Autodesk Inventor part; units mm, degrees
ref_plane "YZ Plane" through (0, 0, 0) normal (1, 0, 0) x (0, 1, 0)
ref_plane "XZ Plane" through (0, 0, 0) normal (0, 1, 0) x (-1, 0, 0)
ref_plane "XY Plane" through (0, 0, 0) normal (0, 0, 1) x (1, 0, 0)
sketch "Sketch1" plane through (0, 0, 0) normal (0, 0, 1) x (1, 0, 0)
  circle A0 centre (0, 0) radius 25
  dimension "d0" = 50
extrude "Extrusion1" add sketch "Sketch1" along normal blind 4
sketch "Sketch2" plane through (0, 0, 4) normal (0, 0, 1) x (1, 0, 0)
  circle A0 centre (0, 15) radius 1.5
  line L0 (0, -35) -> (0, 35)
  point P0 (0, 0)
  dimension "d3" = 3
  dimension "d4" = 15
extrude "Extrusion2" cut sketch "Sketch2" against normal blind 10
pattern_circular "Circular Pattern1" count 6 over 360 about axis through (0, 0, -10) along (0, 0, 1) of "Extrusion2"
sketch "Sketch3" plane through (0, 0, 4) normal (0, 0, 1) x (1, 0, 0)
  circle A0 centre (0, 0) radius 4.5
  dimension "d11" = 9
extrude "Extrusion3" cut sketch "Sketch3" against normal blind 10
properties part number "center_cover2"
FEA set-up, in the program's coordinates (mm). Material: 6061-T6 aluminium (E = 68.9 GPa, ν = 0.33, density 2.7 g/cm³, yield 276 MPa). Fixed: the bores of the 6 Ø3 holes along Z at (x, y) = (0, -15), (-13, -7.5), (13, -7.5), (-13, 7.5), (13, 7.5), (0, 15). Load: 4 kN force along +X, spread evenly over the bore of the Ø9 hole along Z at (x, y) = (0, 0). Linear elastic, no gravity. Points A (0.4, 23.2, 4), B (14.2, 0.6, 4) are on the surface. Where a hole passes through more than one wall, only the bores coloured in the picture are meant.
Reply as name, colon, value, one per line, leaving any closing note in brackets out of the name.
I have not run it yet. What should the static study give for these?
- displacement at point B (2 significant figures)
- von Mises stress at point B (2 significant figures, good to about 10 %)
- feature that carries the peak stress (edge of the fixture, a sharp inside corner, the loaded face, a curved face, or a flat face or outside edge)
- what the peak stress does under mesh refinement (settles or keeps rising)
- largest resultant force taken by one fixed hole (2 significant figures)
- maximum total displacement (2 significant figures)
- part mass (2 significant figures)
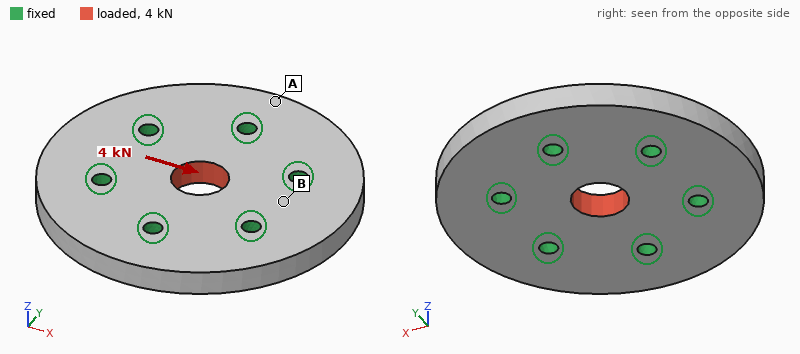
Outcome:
displacement at point B: 1.8 µm
von Mises stress at point B: 11 MPa
feature that carries the peak stress: edge of the fixture
what the peak stress does under mesh refinement: keeps rising
largest resultant force taken by one fixed hole: 900 N
maximum total displacement: 5.0 µm
part mass: 20 g
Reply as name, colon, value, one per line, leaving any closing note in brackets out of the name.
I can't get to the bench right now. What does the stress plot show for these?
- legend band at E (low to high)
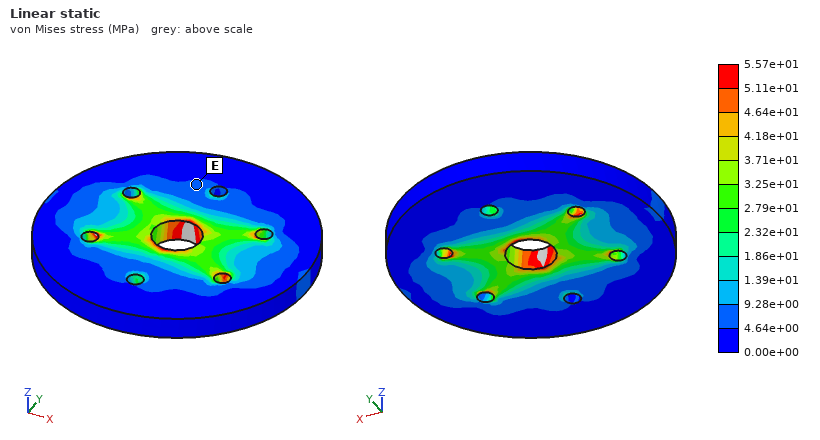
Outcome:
legend band at E: 4.64e+00 to 9.28e+00 MPa
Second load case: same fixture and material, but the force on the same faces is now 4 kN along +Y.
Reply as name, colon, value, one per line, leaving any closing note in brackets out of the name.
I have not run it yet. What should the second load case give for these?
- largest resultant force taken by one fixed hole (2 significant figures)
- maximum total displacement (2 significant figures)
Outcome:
largest resultant force taken by one fixed hole: 1.0 kN
maximum total displacement: 4.9 µm
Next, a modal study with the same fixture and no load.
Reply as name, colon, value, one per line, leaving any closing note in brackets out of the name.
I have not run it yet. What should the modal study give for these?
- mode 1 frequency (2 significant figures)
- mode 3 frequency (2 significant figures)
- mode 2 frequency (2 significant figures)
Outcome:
mode 1 frequency: 24 kHz
mode 3 frequency: 25 kHz
mode 2 frequency: 25 kHz
